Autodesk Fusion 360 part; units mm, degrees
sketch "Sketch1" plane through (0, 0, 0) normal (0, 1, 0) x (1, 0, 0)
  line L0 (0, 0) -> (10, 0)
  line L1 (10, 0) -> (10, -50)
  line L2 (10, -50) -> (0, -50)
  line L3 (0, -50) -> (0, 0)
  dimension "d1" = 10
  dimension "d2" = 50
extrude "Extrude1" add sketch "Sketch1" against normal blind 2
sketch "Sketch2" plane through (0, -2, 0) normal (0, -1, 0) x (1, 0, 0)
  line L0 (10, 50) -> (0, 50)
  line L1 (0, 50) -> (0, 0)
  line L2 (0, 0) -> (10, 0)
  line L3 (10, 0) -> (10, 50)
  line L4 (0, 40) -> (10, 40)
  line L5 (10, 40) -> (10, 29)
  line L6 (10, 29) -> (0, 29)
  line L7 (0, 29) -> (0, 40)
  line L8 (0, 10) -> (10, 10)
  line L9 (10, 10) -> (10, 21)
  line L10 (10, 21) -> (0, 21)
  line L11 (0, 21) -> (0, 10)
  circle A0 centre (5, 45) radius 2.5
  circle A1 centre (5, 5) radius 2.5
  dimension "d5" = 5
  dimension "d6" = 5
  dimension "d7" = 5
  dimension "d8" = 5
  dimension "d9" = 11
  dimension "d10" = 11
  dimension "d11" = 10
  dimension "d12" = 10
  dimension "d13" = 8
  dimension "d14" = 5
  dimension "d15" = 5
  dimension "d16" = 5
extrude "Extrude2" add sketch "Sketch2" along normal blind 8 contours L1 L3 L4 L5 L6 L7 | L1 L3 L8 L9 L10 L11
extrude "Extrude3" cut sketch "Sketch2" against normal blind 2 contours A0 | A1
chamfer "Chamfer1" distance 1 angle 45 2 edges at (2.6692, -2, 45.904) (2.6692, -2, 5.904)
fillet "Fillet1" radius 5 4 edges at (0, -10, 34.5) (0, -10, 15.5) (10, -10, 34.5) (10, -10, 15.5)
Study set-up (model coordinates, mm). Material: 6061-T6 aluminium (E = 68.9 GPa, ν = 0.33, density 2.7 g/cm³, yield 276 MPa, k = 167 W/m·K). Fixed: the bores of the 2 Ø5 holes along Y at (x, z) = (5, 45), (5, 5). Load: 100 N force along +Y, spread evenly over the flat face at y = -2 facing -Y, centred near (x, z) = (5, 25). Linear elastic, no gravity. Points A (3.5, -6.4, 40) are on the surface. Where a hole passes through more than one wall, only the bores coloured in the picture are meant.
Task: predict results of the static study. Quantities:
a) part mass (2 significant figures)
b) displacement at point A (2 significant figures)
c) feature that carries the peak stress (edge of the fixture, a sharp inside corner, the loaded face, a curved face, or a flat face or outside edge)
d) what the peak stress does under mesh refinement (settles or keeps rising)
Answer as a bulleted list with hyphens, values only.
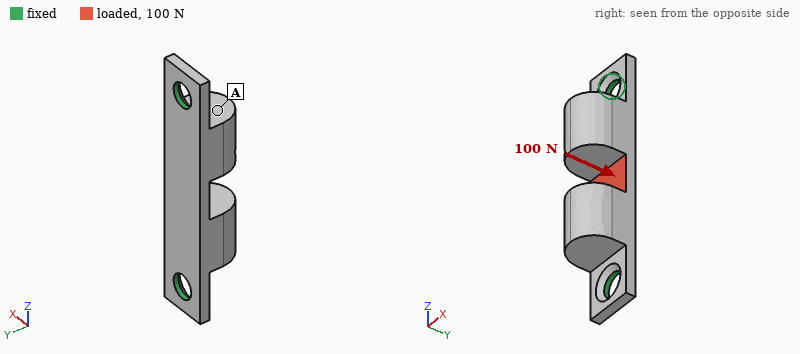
- 6.6 g
- 21 µm
- edge of the fixture
- keeps rising
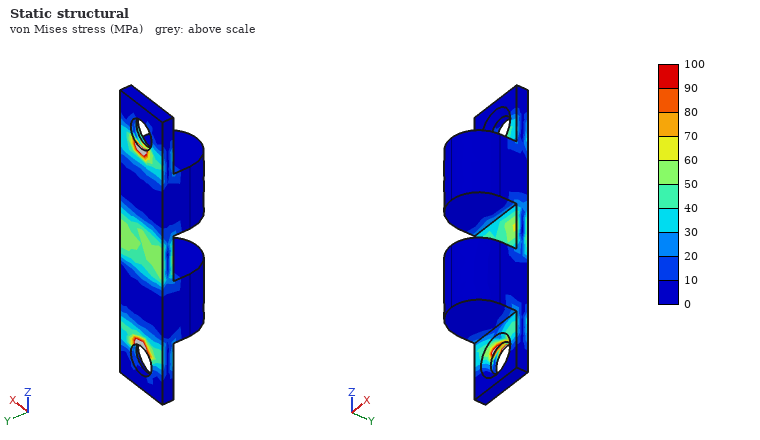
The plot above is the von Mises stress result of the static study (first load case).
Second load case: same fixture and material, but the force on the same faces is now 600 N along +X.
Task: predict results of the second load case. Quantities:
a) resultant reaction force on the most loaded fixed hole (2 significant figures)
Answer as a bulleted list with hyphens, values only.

- 300 N
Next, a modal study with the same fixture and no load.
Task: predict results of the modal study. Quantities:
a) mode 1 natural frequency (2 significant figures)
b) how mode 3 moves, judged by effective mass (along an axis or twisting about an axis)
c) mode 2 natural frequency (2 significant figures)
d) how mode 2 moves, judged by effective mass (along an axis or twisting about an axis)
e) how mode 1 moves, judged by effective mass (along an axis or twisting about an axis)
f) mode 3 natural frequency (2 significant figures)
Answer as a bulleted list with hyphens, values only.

- 4200 Hz
- twisting about Y
- 7800 Hz
- along X
- along Y
- 11 kHz
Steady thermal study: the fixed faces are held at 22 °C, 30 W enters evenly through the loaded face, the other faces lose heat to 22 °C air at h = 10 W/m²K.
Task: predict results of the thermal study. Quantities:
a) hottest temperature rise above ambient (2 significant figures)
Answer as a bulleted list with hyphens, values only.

- 52 K
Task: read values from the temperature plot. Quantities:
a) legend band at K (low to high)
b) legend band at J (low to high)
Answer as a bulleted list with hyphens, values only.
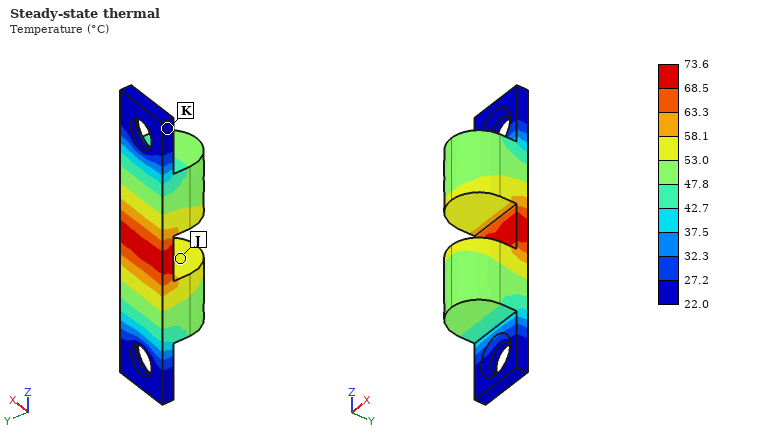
- 22.0 to 27.2 °C
- 53.0 to 58.1 °C
